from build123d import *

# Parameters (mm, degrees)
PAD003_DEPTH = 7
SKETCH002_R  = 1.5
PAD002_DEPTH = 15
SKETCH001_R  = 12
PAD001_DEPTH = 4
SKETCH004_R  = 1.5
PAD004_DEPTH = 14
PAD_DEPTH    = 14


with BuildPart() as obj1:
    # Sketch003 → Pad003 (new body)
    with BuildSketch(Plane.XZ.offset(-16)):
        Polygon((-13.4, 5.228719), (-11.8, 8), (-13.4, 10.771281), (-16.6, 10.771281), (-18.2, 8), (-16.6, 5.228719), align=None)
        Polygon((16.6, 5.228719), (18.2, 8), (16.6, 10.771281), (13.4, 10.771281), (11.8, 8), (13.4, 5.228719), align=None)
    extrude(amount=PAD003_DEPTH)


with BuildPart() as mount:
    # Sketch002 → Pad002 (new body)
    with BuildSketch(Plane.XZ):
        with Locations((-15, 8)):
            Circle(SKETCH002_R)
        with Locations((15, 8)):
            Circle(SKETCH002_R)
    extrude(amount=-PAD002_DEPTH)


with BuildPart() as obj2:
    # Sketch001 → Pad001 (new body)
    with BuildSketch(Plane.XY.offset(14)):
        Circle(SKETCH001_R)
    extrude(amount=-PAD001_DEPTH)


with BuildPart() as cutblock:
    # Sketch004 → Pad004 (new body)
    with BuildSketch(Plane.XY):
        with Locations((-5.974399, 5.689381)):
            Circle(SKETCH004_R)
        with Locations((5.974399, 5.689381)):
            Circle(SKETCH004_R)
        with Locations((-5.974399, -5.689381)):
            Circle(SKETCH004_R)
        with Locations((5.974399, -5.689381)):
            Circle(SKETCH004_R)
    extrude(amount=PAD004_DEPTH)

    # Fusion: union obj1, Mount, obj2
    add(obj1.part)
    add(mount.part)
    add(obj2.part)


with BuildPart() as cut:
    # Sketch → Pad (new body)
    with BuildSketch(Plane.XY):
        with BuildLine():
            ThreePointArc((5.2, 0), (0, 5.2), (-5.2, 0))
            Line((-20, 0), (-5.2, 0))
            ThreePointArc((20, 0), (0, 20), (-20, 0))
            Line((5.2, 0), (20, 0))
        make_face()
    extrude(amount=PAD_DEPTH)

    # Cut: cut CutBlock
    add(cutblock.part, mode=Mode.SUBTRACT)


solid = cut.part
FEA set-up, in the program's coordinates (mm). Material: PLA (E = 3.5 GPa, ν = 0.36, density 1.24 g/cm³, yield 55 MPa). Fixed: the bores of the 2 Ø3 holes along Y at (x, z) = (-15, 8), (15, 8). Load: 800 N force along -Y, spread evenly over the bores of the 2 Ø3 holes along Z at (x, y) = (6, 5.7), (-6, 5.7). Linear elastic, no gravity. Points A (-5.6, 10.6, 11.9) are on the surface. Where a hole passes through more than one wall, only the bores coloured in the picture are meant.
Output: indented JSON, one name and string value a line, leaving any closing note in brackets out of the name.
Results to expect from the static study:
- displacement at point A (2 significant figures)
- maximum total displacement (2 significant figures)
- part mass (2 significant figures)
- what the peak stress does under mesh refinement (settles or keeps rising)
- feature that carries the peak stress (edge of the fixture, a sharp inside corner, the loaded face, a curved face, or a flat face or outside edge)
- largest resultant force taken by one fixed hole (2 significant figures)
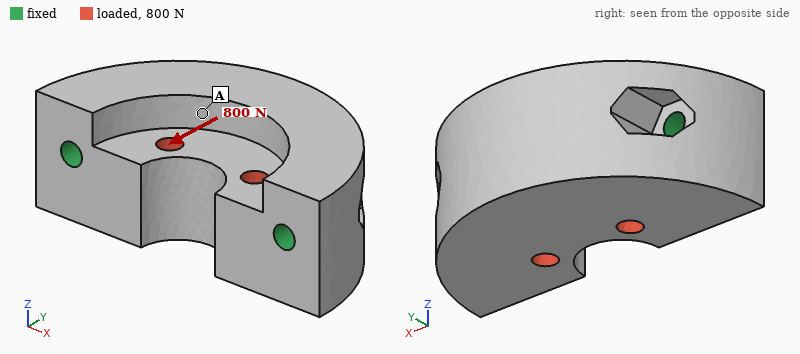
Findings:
{
  "displacement at point A": "18 µm",
  "maximum total displacement": "61 µm",
  "part mass": "8.7 g",
  "what the peak stress does under mesh refinement": "keeps rising",
  "feature that carries the peak stress": "edge of the fixture",
  "largest resultant force taken by one fixed hole": "440 N"
}
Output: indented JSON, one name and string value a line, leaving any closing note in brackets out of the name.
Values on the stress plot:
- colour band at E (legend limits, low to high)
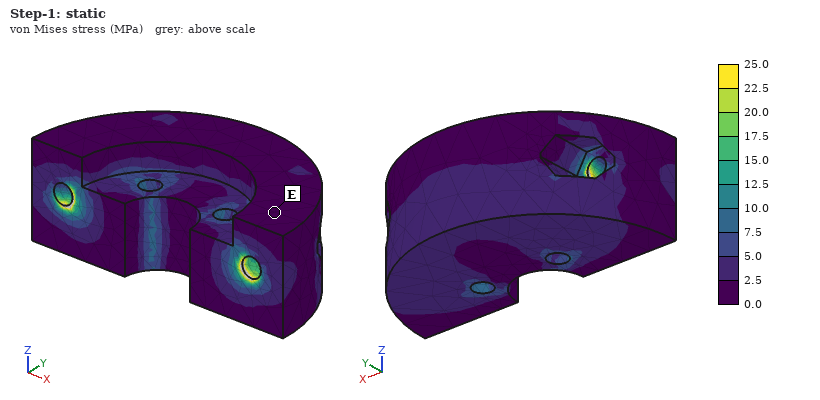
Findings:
{
  "colour band at E": "0.0 to 2.5 MPa"
}
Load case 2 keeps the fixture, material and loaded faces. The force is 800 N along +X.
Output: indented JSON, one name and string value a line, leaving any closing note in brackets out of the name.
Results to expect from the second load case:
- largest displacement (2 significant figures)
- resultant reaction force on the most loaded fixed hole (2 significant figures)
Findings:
{
  "largest displacement": "25 µm",
  "resultant reaction force on the most loaded fixed hole": "410 N"
}
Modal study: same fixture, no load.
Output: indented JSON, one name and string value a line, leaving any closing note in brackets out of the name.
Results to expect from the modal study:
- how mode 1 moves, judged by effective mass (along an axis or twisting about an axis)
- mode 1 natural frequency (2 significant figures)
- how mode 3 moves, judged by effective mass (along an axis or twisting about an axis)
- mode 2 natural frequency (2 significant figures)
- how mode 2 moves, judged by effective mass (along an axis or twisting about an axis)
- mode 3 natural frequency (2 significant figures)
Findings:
{
  "how mode 1 moves, judged by effective mass": "along Z",
  "mode 1 natural frequency": "5600 Hz",
  "how mode 3 moves, judged by effective mass": "along X",
  "mode 2 natural frequency": "11 kHz",
  "how mode 2 moves, judged by effective mass": "along Y",
  "mode 3 natural frequency": "13 kHz"
}
